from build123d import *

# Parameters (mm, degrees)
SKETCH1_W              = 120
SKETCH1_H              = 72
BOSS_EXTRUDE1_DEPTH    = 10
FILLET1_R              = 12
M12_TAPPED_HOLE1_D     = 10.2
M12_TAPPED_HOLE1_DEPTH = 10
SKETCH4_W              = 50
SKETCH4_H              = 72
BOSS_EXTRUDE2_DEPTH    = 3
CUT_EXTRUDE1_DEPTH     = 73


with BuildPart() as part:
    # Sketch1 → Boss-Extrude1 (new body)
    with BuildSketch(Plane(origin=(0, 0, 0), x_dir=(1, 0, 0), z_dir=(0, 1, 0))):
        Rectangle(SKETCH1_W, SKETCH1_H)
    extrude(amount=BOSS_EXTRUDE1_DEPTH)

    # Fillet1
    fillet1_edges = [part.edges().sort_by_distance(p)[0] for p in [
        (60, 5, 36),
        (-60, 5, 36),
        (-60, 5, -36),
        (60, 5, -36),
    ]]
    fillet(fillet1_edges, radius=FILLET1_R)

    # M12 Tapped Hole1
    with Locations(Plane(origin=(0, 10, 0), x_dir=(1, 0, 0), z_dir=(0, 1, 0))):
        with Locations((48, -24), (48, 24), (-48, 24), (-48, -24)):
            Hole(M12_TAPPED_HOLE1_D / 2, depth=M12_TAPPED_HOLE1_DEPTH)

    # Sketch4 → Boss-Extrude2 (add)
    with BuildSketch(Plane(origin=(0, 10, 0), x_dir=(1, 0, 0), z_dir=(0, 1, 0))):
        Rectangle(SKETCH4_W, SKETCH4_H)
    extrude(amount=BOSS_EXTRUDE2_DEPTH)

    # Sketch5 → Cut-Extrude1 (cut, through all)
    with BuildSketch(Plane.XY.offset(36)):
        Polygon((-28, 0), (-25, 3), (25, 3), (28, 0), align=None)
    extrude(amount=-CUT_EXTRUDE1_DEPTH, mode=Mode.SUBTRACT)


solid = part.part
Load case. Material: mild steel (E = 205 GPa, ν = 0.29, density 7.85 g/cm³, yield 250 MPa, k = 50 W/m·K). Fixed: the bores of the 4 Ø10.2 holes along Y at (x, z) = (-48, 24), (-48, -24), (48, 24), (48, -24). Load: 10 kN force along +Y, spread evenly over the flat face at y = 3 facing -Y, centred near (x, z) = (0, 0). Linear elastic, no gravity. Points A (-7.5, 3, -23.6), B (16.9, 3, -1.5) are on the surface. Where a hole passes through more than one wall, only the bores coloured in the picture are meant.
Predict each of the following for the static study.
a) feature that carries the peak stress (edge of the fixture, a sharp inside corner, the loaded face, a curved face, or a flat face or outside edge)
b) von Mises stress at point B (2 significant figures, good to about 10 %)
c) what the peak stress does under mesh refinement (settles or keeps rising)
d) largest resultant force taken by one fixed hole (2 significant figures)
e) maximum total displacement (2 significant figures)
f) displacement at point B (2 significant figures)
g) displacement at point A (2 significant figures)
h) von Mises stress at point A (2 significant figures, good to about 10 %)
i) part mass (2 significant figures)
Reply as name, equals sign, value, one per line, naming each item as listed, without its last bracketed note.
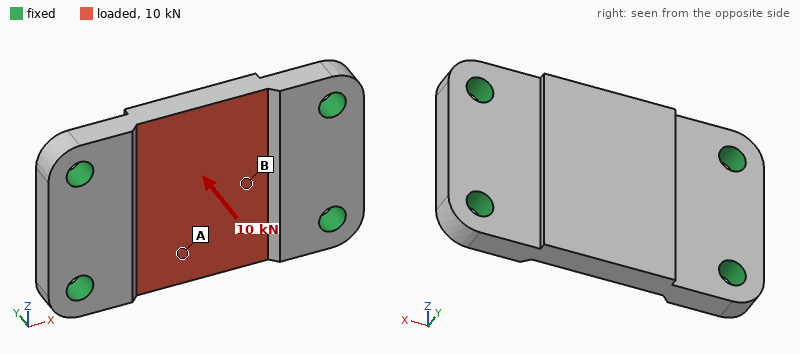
feature that carries the peak stress = edge of the fixture
von Mises stress at point B = 14 MPa
what the peak stress does under mesh refinement = keeps rising
largest resultant force taken by one fixed hole = 3.9 kN
maximum total displacement = 28 µm
displacement at point B = 21 µm
displacement at point A = 26 µm
von Mises stress at point A = 32 MPa
part mass = 640 g
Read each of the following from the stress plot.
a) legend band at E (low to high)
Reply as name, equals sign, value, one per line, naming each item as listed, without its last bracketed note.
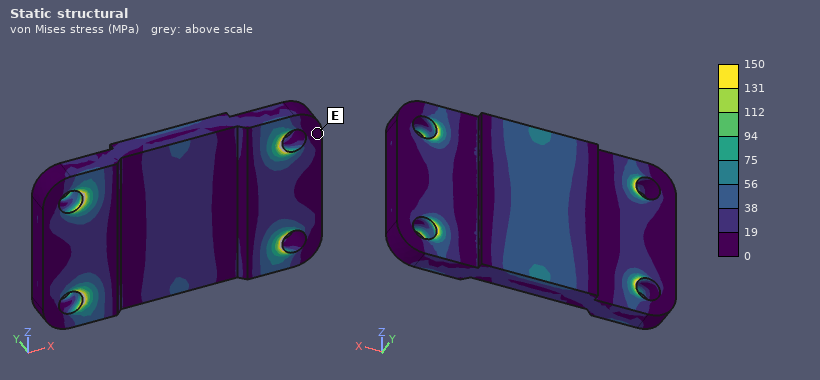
legend band at E = 0 to 19 MPa
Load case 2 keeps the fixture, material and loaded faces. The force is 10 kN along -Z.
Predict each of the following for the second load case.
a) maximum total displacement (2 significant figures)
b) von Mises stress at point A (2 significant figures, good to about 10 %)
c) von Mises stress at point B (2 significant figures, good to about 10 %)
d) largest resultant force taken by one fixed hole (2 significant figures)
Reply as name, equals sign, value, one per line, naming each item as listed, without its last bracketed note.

maximum total displacement = 7.2 µm
von Mises stress at point A = 9.0 MPa
von Mises stress at point B = 17 MPa
largest resultant force taken by one fixed hole = 2.9 kN
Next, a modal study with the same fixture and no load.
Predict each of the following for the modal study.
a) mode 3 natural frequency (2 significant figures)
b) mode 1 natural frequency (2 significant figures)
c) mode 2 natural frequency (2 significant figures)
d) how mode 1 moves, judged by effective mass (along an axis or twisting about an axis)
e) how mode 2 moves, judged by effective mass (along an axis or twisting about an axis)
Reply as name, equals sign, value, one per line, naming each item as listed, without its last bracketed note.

mode 3 natural frequency = 13 kHz
mode 1 natural frequency = 5900 Hz
mode 2 natural frequency = 7600 Hz
how mode 1 moves, judged by effective mass = along Y
how mode 2 moves, judged by effective mass = twisting about X
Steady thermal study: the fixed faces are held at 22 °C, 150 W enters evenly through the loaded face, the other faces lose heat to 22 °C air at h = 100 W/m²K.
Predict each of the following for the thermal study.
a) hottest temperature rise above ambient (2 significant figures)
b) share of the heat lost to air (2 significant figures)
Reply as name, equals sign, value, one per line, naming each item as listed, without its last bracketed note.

hottest temperature rise above ambient = 65 K
share of the heat lost to air = 29 %
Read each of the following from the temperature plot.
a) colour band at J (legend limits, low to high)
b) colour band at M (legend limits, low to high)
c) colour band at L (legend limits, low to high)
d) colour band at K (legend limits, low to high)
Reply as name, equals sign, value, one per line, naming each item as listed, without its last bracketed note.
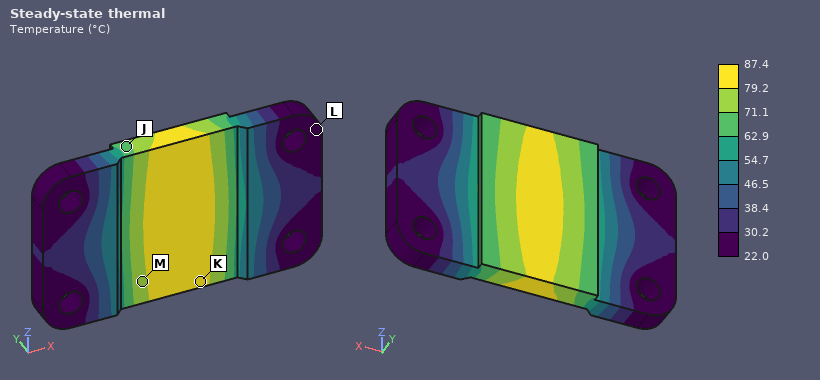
colour band at J = 62.9 to 71.1 °C
colour band at M = 71.1 to 79.2 °C
colour band at L = 22.0 to 30.2 °C
colour band at K = 79.2 to 87.4 °C
